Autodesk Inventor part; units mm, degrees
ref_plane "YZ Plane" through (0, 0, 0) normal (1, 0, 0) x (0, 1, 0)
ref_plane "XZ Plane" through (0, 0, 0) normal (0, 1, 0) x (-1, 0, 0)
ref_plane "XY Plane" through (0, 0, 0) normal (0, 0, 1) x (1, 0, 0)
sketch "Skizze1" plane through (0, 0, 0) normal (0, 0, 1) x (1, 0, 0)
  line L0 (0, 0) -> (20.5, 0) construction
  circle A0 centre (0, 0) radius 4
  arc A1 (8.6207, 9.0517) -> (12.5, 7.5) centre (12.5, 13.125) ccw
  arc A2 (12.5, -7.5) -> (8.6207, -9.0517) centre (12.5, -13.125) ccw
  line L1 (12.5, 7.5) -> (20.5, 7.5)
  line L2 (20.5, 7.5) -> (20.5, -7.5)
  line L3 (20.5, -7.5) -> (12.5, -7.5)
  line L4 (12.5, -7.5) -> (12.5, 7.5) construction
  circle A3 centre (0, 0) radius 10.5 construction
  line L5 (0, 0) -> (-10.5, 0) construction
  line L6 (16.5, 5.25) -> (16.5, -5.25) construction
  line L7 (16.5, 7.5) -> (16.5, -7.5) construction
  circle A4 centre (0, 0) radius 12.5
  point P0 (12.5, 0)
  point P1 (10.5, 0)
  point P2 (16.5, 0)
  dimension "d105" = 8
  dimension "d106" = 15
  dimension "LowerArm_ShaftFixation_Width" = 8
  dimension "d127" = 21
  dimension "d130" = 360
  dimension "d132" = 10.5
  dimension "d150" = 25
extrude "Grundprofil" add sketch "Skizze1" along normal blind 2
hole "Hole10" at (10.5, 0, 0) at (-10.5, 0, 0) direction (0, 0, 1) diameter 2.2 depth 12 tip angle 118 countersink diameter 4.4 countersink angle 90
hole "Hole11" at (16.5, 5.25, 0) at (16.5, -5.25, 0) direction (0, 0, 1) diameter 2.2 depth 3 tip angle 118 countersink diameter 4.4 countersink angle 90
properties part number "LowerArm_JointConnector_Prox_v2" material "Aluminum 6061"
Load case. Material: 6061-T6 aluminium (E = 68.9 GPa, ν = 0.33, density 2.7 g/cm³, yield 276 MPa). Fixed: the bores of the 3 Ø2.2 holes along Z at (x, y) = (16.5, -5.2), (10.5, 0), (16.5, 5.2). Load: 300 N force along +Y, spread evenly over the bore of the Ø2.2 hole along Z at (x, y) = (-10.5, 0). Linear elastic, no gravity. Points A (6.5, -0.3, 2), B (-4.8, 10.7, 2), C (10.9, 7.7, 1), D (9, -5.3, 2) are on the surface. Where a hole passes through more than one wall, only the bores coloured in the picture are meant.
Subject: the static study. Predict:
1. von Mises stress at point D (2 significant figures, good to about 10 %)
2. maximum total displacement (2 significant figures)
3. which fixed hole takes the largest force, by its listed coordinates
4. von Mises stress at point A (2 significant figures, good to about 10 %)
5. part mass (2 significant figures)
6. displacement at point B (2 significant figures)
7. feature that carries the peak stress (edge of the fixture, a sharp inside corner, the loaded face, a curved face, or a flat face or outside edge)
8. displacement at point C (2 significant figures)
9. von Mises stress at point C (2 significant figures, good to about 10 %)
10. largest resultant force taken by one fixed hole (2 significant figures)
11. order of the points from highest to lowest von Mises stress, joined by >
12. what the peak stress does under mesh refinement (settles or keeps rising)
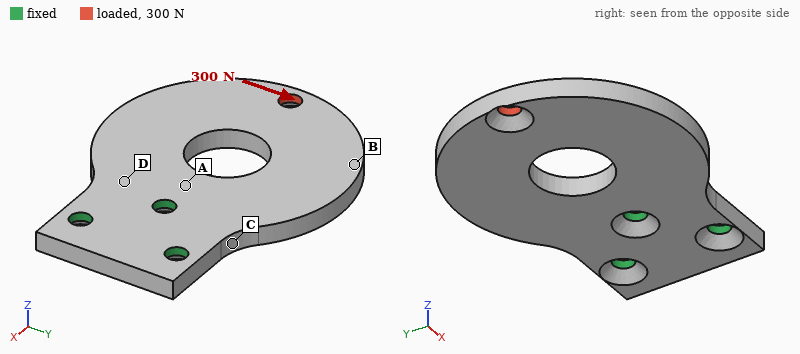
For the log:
36 MPa
60 µm
(10.5, 0)
67 MPa
3.0 g
53 µm
edge of the fixture
10 µm
120 MPa
550 N
C > A > D > B
keeps rising
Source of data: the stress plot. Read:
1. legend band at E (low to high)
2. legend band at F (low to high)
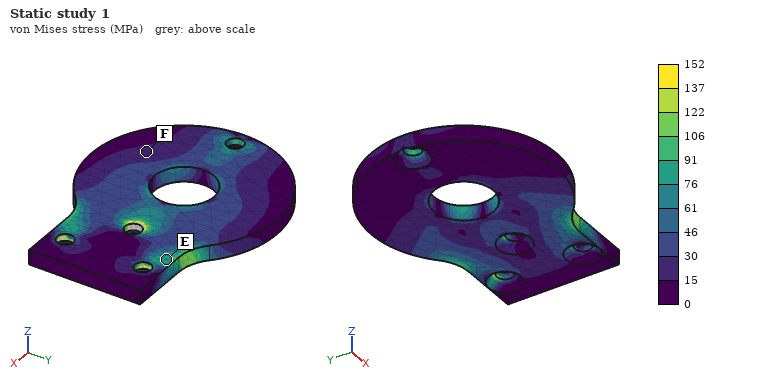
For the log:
76 to 91 MPa
15 to 30 MPa
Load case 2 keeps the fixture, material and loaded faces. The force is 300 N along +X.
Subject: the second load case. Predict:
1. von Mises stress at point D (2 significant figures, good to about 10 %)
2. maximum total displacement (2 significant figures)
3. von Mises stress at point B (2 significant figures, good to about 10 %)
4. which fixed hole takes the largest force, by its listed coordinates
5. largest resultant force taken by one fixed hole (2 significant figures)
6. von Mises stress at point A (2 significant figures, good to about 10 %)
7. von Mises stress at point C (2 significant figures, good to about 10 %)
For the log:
22 MPa
66 µm
8.3 MPa
(10.5, 0)
140 N
14 MPa
21 MPa
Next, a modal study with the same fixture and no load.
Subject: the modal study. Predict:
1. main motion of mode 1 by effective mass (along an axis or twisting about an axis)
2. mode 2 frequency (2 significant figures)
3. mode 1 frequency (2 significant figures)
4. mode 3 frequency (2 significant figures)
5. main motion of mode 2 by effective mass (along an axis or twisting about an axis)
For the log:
along Z
5100 Hz
2800 Hz
12 kHz
twisting about X
